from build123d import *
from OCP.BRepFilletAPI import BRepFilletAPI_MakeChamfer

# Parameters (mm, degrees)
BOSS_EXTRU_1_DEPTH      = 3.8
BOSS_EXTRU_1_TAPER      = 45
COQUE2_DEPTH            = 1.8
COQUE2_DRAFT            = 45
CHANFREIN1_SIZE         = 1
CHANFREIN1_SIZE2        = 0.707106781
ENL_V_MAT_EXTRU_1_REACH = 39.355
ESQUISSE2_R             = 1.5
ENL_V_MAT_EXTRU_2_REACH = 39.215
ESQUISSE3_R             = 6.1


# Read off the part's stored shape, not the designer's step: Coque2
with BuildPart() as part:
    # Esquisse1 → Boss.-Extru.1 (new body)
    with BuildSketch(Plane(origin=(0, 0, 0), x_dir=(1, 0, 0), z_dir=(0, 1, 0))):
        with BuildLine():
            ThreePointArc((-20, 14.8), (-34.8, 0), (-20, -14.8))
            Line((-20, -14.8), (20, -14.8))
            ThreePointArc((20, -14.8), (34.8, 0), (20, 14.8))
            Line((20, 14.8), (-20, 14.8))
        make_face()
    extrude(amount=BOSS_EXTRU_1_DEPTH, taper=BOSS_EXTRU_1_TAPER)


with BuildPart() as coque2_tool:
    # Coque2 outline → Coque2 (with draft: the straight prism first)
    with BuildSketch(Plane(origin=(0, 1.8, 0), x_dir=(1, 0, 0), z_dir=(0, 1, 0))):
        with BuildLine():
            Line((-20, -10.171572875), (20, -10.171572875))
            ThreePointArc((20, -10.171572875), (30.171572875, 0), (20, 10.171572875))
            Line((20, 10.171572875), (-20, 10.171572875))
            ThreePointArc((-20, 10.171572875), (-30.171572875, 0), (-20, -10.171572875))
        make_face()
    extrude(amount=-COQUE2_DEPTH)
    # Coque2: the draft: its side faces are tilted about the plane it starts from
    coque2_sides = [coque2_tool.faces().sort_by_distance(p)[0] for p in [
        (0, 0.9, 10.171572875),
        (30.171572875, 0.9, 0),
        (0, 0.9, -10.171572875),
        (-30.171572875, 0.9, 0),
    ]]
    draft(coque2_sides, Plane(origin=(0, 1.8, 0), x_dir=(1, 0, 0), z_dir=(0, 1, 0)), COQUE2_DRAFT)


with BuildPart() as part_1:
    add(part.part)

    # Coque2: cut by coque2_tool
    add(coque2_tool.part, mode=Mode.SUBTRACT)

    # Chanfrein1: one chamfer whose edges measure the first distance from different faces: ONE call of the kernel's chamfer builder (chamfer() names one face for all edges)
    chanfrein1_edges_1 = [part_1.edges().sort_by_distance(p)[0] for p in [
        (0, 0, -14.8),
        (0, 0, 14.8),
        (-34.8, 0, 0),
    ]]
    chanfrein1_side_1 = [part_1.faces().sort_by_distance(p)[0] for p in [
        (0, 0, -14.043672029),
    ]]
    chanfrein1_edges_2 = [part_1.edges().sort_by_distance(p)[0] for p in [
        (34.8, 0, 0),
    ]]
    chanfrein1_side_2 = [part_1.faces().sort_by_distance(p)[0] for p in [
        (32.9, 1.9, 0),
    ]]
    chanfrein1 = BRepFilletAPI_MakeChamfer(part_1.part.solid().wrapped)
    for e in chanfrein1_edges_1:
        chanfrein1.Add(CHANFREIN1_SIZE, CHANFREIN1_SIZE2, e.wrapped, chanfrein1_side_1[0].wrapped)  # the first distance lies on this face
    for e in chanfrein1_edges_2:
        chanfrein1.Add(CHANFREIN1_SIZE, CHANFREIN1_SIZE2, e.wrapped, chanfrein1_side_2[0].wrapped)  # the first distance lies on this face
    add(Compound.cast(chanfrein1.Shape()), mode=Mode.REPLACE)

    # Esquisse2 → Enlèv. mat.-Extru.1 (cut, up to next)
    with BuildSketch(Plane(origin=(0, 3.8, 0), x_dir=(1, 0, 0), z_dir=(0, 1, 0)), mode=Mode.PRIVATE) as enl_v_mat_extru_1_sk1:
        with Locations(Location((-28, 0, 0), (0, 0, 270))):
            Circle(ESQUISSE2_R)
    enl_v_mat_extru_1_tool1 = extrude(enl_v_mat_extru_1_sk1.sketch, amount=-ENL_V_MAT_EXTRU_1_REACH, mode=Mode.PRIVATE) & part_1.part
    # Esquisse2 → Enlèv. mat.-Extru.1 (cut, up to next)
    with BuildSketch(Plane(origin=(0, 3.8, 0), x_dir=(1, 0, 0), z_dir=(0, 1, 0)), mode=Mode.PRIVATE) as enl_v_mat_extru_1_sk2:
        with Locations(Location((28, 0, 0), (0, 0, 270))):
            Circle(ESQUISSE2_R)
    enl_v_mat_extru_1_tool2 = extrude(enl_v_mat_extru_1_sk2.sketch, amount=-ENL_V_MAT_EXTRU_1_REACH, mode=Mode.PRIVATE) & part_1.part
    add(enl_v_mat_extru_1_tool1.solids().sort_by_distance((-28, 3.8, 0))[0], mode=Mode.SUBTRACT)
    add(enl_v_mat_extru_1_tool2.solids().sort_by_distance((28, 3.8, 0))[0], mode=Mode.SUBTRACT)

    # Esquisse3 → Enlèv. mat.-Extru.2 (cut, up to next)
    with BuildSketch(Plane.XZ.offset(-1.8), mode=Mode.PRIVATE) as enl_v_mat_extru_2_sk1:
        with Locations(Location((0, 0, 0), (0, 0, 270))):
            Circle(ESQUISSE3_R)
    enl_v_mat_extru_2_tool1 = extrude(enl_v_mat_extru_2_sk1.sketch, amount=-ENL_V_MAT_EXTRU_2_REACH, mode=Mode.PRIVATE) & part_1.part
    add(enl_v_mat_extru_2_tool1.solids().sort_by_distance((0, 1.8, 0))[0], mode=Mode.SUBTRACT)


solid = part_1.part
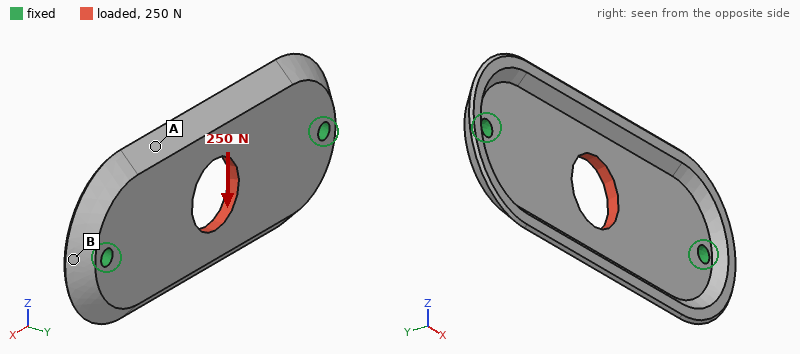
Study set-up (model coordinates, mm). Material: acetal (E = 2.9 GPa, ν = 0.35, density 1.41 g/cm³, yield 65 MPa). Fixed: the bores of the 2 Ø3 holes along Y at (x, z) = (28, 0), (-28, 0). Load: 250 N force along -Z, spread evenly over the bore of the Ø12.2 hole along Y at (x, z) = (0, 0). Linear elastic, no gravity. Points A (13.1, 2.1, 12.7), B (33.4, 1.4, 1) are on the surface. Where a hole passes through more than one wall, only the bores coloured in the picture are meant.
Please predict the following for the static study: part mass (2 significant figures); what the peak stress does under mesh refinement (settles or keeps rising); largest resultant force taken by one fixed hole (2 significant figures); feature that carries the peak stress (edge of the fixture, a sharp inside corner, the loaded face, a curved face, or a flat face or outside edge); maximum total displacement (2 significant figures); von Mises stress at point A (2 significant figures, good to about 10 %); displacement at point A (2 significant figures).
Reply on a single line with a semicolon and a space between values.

4.7 g; keeps rising; 130 N; edge of the fixture; 0.27 mm; 5.7 MPa; 0.16 mm
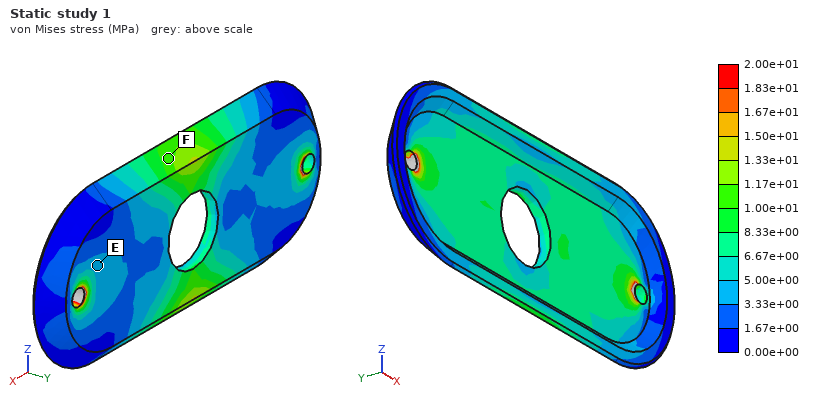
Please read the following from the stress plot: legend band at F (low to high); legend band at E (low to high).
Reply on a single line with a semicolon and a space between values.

1.00e+01 to 1.17e+01 MPa; 3.33e+00 to 5.00e+00 MPa
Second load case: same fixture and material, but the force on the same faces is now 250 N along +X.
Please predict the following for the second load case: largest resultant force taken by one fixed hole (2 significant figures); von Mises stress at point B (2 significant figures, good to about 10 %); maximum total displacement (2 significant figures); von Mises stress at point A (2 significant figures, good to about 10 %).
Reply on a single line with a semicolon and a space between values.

130 N; 3.4 MPa; 38 µm; 1.2 MPa
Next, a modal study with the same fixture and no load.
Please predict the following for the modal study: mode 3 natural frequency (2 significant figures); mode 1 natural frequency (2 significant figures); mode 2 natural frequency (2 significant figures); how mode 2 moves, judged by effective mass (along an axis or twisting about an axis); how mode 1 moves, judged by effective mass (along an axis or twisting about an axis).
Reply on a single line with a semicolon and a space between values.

2400 Hz; 1100 Hz; 1200 Hz; twisting about X; along Y
